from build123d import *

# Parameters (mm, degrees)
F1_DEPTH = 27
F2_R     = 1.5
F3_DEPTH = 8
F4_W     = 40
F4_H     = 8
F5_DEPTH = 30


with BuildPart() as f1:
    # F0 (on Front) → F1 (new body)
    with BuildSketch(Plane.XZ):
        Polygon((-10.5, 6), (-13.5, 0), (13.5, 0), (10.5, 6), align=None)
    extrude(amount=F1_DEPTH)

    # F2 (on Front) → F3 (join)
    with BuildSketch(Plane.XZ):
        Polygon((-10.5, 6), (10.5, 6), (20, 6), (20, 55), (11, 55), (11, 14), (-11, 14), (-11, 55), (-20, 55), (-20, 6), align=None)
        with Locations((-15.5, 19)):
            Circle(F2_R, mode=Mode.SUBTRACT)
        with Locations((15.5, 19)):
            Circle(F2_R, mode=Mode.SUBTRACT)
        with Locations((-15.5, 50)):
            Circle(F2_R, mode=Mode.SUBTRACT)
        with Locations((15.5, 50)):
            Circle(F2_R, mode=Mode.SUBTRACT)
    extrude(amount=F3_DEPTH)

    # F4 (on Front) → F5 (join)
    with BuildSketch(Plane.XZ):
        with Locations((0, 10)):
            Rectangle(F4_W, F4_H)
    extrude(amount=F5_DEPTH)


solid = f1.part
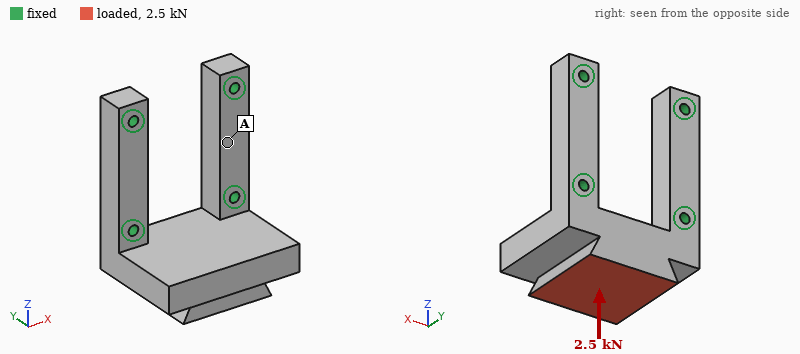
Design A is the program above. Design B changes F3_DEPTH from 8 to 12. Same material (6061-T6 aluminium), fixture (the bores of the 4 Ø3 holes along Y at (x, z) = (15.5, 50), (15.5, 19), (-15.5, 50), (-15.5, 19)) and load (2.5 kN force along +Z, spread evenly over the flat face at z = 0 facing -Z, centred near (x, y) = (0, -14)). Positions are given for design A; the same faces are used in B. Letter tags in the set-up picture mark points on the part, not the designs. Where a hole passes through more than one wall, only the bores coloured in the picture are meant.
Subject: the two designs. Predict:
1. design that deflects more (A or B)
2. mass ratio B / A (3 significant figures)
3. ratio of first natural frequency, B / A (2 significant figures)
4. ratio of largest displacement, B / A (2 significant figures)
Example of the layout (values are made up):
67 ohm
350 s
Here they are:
A
1.15
1.7
0.31
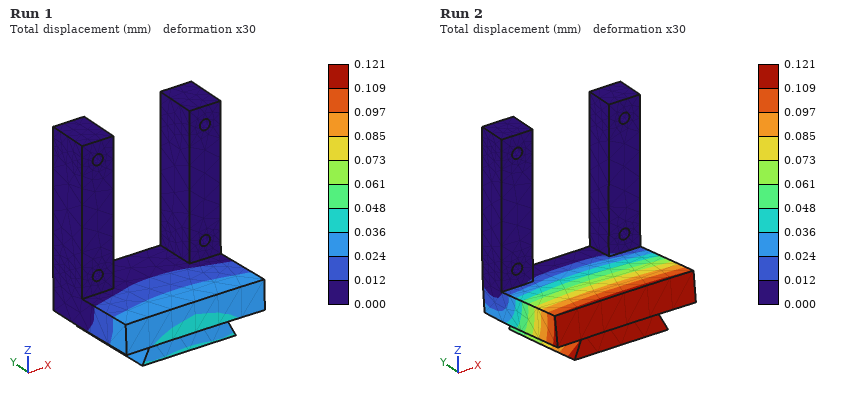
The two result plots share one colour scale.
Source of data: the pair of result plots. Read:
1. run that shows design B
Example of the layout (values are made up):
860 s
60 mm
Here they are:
Run 1
